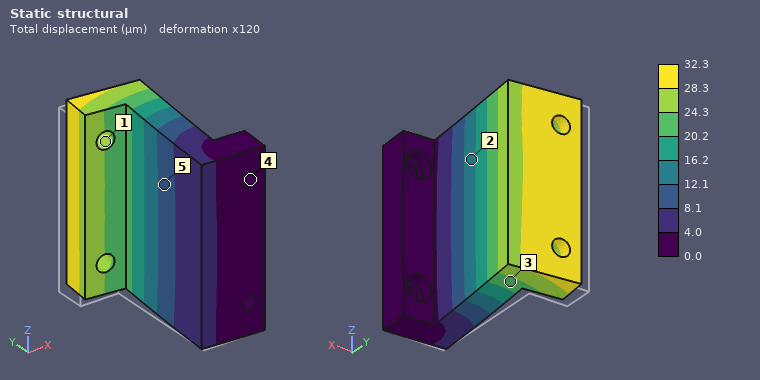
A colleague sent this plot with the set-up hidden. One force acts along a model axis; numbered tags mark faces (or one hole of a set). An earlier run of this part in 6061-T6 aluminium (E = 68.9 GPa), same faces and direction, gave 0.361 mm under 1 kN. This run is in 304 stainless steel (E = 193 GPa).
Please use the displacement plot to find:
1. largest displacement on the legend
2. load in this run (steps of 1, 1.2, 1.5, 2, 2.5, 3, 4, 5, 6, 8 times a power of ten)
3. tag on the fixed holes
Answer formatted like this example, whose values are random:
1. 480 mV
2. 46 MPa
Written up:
1. 32.3 µm
2. 250 N
3. 4
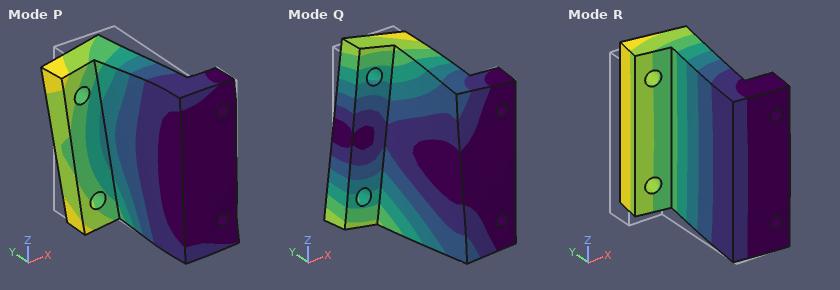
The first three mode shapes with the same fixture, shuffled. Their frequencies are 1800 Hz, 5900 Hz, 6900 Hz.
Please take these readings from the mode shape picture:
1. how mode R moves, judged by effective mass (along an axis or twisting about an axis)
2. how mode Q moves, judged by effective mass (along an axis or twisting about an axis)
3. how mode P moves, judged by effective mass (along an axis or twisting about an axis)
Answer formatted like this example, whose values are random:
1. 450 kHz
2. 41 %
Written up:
1. along X
2. along Z
3. along Z
